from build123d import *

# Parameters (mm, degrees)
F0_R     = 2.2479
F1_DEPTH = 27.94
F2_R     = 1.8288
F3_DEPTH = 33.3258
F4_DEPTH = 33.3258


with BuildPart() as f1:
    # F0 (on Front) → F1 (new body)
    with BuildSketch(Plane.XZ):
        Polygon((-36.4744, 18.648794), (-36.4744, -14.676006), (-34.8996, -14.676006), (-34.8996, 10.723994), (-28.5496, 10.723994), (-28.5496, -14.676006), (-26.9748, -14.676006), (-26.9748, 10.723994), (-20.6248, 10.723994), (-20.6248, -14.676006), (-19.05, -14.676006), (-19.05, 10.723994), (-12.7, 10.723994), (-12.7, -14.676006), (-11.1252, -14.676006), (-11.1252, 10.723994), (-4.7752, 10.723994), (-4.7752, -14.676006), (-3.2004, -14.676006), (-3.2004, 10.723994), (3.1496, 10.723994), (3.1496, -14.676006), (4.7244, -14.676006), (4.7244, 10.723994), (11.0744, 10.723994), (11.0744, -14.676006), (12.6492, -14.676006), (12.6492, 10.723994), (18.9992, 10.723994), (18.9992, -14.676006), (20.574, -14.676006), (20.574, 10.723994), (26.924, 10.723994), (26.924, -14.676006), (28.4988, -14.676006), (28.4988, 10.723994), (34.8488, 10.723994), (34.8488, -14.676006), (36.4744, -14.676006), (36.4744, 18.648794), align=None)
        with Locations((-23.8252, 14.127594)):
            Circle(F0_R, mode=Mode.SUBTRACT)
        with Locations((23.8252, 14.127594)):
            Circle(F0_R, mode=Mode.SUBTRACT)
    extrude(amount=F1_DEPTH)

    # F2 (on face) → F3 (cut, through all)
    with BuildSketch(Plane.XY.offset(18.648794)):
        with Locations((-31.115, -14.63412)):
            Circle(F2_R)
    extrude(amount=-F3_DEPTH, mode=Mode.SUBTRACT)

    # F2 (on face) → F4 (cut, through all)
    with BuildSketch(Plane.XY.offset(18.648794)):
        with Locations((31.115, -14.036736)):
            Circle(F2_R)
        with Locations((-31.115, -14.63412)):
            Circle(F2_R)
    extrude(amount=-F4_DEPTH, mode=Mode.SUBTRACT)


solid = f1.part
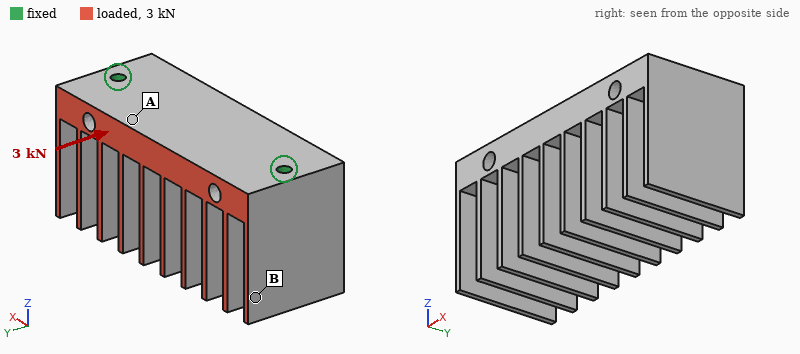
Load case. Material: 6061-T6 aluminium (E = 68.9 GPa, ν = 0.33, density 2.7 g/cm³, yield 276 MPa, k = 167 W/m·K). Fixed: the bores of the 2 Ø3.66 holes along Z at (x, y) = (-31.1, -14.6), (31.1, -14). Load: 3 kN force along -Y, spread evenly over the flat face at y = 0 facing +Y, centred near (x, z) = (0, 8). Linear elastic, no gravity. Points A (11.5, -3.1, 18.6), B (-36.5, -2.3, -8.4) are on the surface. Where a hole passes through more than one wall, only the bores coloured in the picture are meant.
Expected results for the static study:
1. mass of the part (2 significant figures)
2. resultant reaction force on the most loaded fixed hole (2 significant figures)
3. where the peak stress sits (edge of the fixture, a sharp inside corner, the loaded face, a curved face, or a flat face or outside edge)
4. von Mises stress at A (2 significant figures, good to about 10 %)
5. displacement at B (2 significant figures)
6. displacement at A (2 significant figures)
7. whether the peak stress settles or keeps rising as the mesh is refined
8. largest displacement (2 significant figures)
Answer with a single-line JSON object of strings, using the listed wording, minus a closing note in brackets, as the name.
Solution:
{"mass of the part": "71 g", "resultant reaction force on the most loaded fixed hole": "1.5 kN", "where the peak stress sits": "edge of the fixture", "von Mises stress at A": "15 MPa", "displacement at B": "19 µm", "displacement at A": "19 µm", "whether the peak stress settles or keeps rising as the mesh is refined": "keeps rising", "largest displacement": "77 µm"}
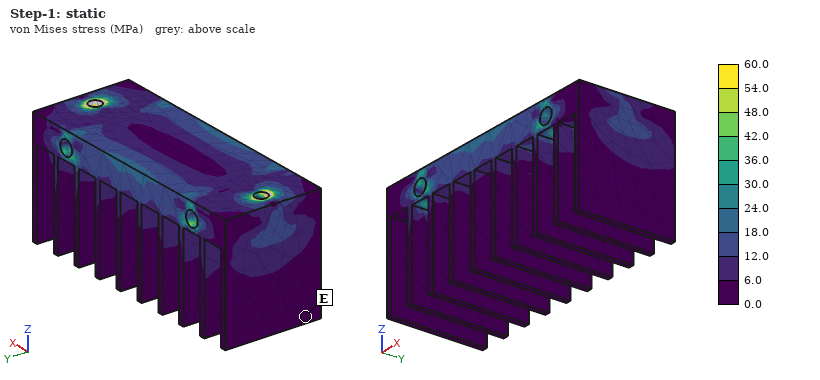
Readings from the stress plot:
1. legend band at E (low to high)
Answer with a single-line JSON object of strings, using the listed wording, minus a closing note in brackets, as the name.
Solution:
{"legend band at E": "0.0 to 6.0 MPa"}
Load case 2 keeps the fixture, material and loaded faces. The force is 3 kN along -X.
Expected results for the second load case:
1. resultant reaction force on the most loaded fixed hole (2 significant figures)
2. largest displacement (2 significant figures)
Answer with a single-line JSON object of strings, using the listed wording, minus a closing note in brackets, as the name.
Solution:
{"resultant reaction force on the most loaded fixed hole": "1.7 kN", "largest displacement": "0.67 mm"}
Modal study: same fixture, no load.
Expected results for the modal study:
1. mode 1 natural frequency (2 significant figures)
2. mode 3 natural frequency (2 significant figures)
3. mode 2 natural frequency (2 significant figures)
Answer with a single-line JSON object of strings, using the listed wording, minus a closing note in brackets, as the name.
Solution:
{"mode 1 natural frequency": "1900 Hz", "mode 3 natural frequency": "2000 Hz", "mode 2 natural frequency": "2000 Hz"}
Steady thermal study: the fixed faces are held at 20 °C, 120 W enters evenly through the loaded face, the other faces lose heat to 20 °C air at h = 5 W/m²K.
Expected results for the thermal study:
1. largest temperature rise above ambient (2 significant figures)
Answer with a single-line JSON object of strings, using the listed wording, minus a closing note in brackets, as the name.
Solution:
{"largest temperature rise above ambient": "49 K"}
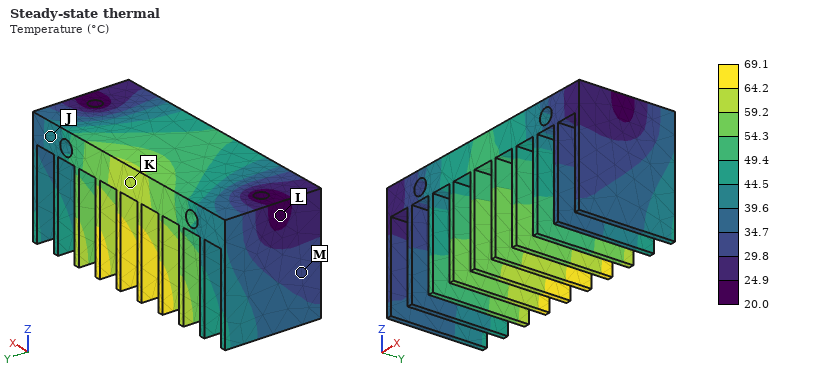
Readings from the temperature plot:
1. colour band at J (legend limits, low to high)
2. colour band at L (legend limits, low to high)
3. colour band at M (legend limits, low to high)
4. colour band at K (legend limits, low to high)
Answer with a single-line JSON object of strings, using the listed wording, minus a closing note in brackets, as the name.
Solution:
{"colour band at J": "39.6 to 44.5 °C", "colour band at L": "20.0 to 24.9 °C", "colour band at M": "29.8 to 34.7 °C", "colour band at K": "59.2 to 64.2 °C"}
